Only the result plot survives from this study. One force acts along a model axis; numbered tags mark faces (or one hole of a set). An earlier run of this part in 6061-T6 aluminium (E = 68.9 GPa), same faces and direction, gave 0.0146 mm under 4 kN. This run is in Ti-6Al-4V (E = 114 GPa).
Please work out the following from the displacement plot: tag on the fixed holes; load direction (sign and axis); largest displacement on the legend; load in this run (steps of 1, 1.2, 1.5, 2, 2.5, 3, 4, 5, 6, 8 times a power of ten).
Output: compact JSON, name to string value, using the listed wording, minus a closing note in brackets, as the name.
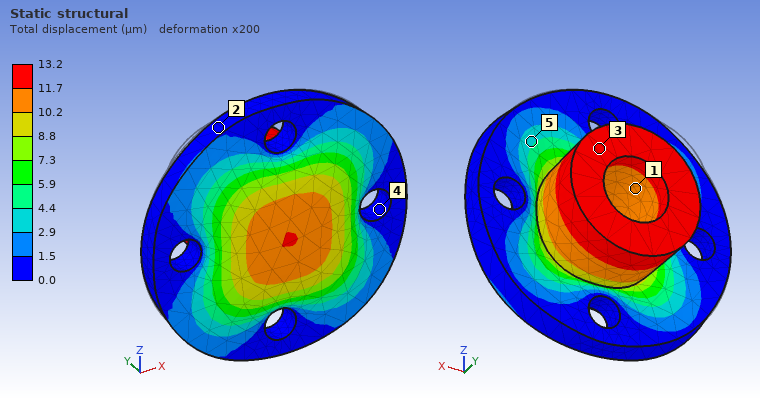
{"tag on the fixed holes": "4", "load direction": "-Y", "largest displacement on the legend": "13.2 µm", "load in this run": "6 kN"}
